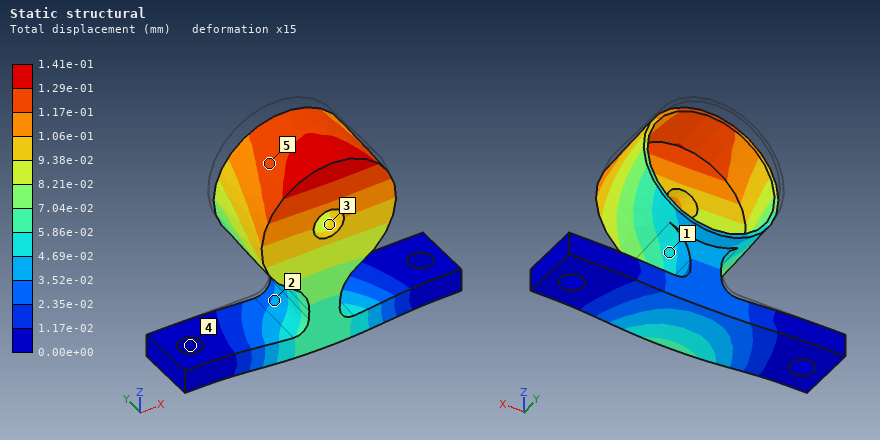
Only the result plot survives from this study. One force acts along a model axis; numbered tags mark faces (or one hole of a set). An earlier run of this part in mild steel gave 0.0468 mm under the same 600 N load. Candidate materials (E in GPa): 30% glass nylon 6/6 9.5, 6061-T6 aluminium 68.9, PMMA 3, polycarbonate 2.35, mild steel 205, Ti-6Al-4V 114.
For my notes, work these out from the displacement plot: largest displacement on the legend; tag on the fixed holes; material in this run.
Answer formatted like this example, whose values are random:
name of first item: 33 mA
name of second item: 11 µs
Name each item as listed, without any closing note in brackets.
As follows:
largest displacement on the legend: 1.41e-01 mm
tag on the fixed holes: 4
material in this run: 6061-T6 aluminium
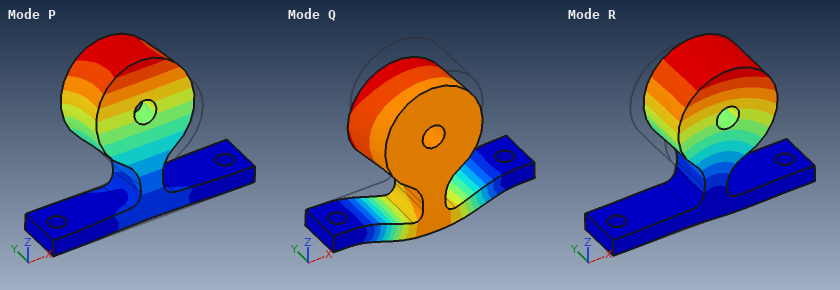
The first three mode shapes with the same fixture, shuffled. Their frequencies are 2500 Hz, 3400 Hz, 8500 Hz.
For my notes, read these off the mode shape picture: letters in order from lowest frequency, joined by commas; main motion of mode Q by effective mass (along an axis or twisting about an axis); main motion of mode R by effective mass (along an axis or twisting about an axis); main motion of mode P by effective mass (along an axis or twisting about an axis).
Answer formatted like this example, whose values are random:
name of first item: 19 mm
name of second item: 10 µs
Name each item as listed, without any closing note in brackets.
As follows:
letters in order from lowest frequency, joined by commas: P, R, Q
main motion of mode Q by effective mass: along Z
main motion of mode R by effective mass: along X
main motion of mode P by effective mass: along Y
